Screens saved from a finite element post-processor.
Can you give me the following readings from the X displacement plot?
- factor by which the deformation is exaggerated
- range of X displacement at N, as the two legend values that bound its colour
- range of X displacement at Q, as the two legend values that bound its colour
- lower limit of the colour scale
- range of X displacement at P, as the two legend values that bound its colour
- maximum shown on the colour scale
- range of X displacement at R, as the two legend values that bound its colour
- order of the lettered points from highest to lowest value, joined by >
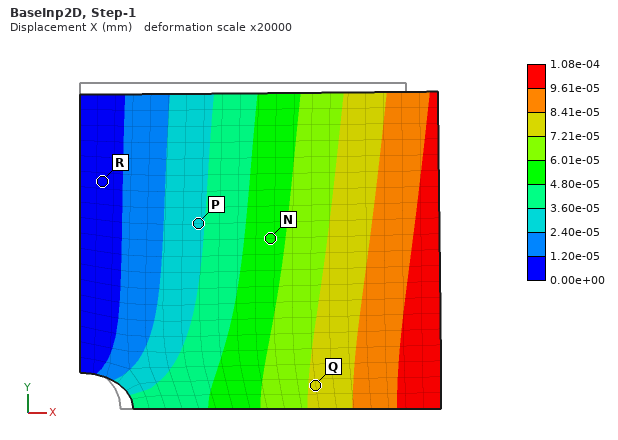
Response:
20000
4.80e-05 to 6.01e-05 mm
7.21e-05 to 8.41e-05 mm
0.00e+00 mm
2.40e-05 to 3.60e-05 mm
1.08e-04 mm
0.00e+00 to 1.20e-05 mm
Q > N > P > R
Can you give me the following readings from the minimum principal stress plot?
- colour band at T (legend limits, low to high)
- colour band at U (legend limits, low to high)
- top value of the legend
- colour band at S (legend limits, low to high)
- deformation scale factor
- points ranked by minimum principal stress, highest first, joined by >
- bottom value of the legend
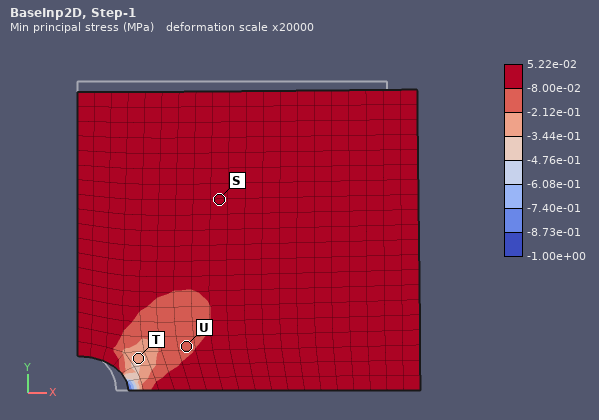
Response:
-3.44e-01 to -2.12e-01 MPa
-2.12e-01 to -8.00e-02 MPa
5.22e-02 MPa
-8.00e-02 to 5.22e-02 MPa
20000
S > U > T
-1.00e+00 MPa
